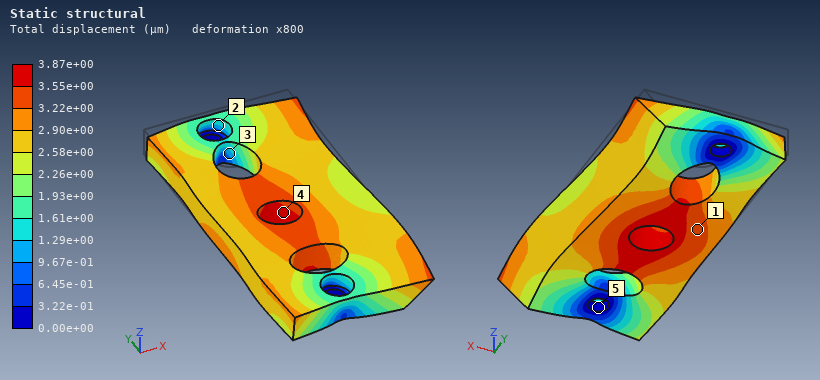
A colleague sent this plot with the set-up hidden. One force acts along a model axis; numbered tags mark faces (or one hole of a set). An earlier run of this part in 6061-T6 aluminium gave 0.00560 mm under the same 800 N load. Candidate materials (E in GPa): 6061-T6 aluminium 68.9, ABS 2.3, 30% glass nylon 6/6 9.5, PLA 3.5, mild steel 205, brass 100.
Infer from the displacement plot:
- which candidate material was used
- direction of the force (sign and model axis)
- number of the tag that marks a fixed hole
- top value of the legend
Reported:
brass
-Y
5
3.87e+00 µm
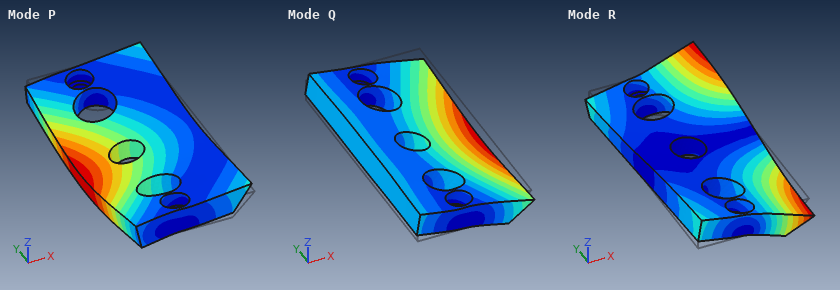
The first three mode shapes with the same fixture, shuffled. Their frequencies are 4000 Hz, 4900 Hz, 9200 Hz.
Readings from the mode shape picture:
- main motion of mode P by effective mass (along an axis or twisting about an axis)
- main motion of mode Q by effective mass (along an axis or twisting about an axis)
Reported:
along Z
along Z
